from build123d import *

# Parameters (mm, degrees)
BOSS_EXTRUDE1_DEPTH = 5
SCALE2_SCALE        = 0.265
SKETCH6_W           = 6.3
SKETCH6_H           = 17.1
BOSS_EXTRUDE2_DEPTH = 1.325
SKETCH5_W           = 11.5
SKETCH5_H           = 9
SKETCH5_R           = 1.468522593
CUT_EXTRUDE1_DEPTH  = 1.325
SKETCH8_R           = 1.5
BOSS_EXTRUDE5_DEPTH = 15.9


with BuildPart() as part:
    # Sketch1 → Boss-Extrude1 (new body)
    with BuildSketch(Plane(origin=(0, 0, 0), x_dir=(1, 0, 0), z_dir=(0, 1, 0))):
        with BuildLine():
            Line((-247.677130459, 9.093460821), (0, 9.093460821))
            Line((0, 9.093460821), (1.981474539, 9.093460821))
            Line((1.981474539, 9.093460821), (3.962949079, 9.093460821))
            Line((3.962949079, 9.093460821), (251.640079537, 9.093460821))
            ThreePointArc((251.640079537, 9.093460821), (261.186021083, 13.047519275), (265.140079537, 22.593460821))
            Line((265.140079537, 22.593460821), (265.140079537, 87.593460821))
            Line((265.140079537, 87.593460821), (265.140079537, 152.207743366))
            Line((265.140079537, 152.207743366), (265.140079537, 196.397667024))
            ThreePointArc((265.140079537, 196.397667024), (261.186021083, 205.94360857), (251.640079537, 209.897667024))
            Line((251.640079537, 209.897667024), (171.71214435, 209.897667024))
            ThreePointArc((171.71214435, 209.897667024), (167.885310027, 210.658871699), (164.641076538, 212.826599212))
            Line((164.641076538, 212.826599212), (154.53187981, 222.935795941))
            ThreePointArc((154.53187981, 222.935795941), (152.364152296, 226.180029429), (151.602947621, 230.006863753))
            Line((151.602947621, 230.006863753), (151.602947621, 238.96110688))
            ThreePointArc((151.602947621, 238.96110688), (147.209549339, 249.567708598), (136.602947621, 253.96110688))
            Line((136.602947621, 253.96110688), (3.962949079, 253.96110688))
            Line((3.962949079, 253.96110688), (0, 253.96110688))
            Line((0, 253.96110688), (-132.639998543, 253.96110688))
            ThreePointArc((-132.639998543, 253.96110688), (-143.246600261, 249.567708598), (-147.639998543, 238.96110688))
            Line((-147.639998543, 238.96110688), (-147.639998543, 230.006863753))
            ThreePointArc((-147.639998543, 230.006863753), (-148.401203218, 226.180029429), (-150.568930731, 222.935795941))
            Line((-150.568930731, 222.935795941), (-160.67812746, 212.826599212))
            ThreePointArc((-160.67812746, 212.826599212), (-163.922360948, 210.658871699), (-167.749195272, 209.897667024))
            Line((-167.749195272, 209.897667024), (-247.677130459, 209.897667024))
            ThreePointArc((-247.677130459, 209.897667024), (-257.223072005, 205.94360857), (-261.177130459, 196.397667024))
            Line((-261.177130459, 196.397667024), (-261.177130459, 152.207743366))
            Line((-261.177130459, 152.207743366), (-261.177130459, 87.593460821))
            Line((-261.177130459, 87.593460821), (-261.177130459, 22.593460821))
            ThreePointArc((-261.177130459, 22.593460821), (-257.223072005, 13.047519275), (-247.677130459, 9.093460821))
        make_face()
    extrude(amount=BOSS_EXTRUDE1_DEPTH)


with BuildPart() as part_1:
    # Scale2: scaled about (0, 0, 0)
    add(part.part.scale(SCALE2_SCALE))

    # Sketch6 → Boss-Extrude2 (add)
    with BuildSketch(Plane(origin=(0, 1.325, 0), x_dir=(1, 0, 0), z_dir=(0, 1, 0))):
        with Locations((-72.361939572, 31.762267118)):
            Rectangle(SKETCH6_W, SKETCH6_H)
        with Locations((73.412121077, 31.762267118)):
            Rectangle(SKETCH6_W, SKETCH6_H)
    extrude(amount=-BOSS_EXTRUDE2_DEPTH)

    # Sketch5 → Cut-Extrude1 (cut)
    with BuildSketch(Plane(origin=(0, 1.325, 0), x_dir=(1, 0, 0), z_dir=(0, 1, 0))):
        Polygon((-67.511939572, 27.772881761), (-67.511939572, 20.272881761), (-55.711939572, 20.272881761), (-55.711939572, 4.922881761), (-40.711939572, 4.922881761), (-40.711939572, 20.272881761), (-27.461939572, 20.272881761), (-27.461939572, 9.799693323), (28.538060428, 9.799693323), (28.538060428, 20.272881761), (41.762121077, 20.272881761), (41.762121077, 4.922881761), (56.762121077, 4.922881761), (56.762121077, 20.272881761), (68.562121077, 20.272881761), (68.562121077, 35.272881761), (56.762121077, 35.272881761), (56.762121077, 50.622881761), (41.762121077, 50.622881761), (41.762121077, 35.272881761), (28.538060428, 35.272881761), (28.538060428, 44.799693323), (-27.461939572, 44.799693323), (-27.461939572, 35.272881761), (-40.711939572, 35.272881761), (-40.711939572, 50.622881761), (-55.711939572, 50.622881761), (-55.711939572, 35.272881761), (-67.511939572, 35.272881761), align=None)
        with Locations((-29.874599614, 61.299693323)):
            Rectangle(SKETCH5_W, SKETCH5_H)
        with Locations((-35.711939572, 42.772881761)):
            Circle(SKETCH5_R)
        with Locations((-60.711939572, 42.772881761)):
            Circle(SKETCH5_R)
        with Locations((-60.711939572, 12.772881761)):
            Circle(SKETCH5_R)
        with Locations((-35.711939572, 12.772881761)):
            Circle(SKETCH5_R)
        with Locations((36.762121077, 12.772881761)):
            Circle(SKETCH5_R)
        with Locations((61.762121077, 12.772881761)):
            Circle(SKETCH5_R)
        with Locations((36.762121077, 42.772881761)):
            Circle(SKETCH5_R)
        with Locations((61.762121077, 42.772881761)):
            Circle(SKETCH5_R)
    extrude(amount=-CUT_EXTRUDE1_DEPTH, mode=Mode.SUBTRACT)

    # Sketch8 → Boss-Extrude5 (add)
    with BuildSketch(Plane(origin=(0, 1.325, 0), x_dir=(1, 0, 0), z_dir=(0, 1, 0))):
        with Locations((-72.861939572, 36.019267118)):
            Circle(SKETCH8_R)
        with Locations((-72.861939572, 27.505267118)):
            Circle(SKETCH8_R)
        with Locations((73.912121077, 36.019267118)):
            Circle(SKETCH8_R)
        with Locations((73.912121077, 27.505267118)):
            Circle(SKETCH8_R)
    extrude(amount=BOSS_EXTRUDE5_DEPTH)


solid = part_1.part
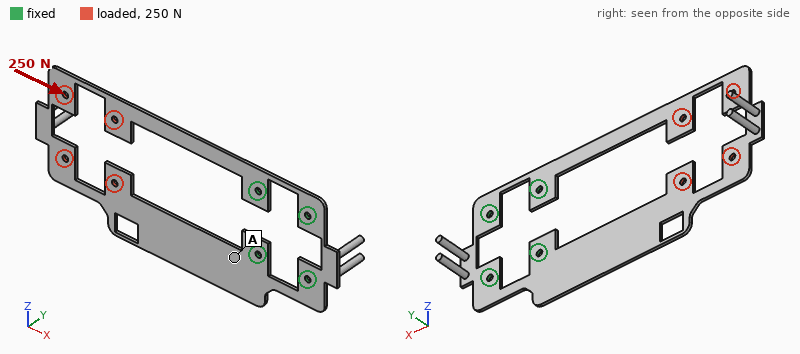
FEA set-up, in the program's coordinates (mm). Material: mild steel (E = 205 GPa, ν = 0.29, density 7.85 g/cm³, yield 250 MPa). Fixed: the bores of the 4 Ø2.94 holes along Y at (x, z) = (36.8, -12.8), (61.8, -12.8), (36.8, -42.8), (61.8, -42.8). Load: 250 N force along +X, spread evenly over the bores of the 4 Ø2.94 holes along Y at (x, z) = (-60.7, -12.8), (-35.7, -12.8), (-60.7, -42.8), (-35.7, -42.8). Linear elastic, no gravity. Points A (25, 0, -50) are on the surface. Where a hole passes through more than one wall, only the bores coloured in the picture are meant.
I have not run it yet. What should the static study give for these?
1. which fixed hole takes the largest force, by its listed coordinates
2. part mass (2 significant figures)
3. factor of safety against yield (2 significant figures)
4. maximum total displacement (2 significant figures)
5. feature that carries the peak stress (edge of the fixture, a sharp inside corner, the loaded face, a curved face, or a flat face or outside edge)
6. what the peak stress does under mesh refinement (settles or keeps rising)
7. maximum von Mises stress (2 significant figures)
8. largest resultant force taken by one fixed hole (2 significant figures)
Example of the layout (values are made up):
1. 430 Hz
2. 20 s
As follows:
1. (36.8, -42.8)
2. 49 g
3. 1.0
4. 0.13 mm
5. a flat face or outside edge
6. settles
7. 250 MPa
8. 79 N
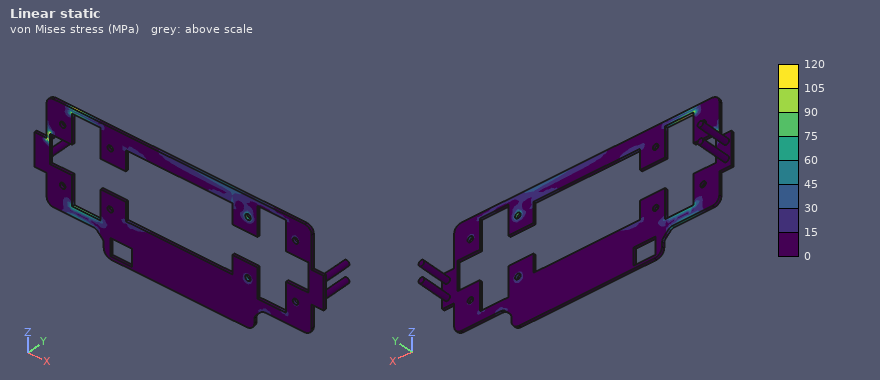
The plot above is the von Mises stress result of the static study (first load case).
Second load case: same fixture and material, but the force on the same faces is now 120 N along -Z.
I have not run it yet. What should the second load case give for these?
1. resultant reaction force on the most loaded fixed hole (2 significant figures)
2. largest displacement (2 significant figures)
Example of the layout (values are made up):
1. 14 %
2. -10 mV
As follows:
1. 380 N
2. 0.38 mm
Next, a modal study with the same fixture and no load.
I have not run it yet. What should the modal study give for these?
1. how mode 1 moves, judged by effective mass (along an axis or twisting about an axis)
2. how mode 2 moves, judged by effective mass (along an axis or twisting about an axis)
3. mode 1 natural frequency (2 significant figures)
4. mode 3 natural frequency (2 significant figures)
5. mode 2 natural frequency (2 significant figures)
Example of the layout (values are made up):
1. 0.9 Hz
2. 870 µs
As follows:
1. along Y
2. twisting about X
3. 79 Hz
4. 390 Hz
5. 230 Hz
